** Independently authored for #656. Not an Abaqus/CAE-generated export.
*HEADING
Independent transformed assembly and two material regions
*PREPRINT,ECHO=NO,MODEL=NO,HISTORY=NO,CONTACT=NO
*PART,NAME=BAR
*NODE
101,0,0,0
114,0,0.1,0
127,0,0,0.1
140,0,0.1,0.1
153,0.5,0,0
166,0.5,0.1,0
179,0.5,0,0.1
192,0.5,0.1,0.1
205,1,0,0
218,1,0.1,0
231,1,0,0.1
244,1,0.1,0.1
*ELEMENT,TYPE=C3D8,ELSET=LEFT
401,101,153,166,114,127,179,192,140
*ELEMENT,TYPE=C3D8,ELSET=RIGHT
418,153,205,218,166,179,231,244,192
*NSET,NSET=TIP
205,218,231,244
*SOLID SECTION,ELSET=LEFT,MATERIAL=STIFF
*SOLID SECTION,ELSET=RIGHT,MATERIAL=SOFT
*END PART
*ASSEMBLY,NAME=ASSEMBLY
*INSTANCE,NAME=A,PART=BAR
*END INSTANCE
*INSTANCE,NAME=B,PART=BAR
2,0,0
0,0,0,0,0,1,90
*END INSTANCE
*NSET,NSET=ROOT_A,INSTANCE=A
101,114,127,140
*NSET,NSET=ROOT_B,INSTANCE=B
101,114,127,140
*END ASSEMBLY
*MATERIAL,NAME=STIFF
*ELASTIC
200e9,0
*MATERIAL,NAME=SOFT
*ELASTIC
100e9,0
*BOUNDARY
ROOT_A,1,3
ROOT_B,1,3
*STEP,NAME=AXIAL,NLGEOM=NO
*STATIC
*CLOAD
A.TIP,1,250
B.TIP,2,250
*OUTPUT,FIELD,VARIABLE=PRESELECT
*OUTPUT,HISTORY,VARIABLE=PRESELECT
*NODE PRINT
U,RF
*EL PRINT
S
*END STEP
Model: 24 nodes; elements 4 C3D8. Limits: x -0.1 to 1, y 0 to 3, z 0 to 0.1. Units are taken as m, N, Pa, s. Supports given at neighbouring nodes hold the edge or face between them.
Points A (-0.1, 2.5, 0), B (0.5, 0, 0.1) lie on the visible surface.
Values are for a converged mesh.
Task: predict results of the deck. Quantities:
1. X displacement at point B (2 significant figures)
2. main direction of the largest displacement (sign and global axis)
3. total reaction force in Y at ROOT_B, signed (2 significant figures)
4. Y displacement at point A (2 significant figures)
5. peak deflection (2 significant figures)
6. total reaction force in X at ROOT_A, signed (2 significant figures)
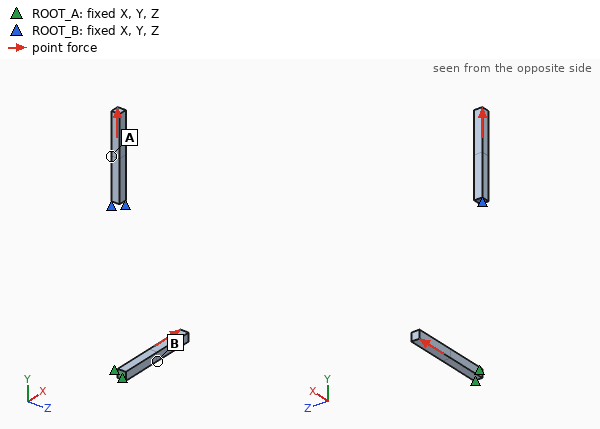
2.5e-07 m
+X
-1000 N
2.5e-07 m
7.7e-07 m
-1000 N
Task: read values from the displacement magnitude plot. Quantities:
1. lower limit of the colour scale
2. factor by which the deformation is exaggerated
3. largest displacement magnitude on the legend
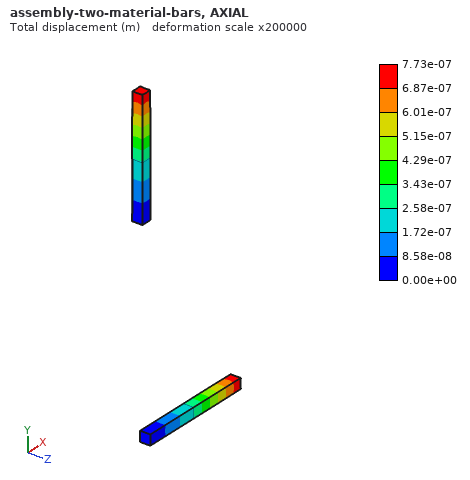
0.00e+00 m
200000
7.73e-07 m
